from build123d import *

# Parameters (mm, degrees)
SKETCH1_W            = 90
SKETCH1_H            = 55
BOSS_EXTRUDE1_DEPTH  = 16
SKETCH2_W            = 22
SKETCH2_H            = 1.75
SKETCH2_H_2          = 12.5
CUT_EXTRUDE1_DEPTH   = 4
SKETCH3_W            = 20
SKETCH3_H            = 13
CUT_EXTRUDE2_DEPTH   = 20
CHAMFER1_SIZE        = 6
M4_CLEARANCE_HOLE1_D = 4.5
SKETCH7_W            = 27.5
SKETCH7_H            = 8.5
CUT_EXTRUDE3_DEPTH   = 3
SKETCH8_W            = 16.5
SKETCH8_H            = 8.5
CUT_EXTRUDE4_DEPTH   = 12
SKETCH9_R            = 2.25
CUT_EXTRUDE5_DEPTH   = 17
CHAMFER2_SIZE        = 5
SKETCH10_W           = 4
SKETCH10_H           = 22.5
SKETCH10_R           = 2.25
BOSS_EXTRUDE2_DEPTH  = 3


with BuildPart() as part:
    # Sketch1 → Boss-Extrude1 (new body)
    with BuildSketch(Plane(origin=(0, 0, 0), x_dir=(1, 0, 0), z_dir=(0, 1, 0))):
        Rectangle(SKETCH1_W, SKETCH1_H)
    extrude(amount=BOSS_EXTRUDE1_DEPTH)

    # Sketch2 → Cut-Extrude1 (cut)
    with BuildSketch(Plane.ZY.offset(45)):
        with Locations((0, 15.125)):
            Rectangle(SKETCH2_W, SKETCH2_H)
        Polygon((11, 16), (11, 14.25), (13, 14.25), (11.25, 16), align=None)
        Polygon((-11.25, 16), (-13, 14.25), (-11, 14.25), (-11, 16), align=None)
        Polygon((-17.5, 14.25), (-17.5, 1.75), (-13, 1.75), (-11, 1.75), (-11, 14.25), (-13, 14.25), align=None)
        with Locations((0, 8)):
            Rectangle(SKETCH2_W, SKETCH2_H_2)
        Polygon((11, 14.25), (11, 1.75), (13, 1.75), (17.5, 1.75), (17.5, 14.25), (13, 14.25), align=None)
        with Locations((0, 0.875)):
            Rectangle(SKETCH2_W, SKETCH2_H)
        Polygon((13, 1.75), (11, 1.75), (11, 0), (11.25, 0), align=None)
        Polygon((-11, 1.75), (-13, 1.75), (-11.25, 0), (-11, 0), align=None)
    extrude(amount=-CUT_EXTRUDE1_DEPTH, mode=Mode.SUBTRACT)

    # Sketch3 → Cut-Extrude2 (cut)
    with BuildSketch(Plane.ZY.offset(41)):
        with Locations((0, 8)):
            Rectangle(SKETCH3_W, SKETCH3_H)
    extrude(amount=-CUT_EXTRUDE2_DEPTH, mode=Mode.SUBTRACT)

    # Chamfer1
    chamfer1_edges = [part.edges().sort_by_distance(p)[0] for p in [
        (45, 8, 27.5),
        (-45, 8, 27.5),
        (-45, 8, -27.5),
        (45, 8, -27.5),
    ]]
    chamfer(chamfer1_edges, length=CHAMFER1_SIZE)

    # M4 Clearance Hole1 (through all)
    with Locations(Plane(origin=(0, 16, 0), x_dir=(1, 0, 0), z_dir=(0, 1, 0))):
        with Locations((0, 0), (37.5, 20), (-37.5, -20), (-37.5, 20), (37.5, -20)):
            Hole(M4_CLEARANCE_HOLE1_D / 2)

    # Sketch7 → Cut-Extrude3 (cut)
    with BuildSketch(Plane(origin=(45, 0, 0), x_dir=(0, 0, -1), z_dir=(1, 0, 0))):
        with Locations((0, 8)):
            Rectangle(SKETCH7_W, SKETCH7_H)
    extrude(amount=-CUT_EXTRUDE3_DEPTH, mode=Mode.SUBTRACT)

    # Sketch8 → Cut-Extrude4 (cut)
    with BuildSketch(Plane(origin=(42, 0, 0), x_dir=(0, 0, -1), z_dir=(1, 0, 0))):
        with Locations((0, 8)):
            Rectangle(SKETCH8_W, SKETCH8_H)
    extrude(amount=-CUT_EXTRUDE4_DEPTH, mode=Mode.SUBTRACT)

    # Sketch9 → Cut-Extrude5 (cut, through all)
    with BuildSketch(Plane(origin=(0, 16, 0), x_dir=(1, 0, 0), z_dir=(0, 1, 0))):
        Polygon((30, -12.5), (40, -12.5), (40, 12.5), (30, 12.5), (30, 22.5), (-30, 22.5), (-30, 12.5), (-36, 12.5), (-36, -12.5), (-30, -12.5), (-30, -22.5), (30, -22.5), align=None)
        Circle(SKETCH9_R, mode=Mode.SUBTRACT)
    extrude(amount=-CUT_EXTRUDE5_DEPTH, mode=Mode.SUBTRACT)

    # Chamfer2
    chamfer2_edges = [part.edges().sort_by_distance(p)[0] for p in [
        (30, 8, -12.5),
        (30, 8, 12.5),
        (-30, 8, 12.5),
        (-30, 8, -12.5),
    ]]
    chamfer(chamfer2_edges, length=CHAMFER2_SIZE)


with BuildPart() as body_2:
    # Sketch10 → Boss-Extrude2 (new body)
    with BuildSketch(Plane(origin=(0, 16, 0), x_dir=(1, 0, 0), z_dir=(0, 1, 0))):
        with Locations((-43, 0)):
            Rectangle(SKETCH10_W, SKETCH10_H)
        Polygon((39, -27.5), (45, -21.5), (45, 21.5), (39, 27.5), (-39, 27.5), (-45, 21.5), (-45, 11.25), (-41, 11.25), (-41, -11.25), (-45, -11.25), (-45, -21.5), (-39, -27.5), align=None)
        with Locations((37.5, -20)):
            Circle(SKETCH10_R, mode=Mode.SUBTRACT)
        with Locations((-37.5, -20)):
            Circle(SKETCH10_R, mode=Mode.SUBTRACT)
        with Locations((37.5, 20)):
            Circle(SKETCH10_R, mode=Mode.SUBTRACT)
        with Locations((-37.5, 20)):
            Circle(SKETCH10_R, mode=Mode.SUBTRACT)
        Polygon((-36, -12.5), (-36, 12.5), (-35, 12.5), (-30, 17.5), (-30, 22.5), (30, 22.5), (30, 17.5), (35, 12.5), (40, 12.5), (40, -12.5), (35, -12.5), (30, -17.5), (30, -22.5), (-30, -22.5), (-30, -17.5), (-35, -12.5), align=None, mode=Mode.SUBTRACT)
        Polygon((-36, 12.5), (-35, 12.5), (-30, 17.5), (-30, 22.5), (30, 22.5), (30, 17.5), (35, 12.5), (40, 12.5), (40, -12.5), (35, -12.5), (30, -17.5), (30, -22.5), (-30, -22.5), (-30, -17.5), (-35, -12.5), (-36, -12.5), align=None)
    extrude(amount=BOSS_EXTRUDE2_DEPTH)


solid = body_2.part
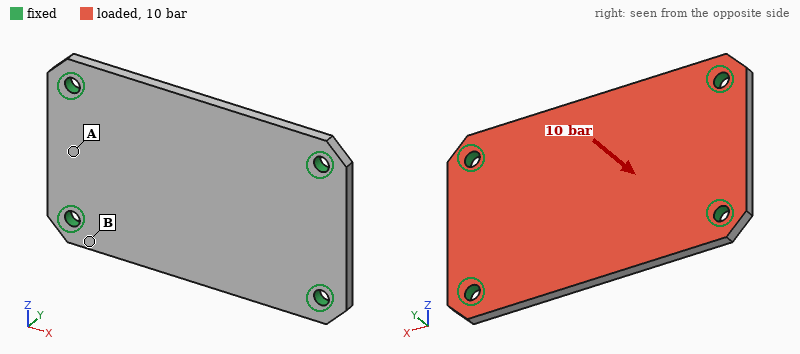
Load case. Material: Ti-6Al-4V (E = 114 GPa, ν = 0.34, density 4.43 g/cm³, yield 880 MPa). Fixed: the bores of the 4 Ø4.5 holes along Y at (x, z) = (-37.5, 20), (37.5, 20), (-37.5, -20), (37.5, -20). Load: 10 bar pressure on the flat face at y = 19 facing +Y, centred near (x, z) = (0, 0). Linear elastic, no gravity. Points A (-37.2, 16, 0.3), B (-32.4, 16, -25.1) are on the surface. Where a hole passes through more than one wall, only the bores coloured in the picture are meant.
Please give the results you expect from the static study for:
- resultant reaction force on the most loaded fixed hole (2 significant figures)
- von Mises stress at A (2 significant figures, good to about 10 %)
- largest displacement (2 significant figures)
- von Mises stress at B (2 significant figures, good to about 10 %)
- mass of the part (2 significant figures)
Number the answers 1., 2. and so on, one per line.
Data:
1. 1.2 kN
2. 73 MPa
3. 0.35 mm
4. 230 MPa
5. 64 g
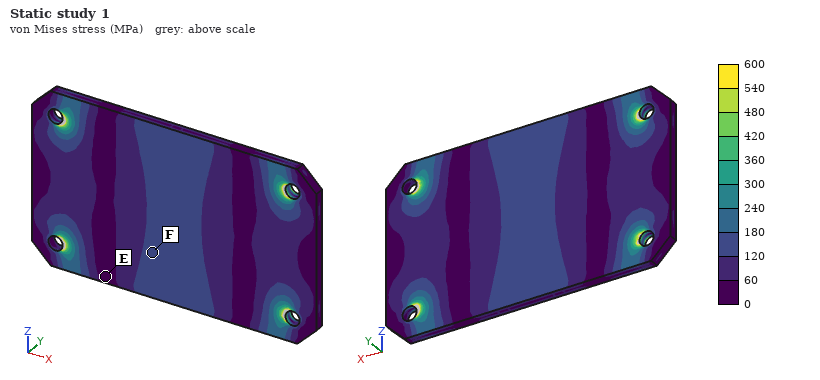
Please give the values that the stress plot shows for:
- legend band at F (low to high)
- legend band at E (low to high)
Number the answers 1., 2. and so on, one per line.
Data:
1. 120 to 180 MPa
2. 0 to 60 MPa
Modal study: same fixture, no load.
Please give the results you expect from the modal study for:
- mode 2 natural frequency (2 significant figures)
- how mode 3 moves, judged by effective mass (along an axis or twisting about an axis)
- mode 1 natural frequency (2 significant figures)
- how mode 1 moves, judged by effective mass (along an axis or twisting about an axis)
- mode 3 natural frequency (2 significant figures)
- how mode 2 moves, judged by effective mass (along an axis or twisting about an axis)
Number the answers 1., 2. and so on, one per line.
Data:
1. 3800 Hz
2. twisting about Z
3. 2600 Hz
4. along Y
5. 7000 Hz
6. twisting about X
